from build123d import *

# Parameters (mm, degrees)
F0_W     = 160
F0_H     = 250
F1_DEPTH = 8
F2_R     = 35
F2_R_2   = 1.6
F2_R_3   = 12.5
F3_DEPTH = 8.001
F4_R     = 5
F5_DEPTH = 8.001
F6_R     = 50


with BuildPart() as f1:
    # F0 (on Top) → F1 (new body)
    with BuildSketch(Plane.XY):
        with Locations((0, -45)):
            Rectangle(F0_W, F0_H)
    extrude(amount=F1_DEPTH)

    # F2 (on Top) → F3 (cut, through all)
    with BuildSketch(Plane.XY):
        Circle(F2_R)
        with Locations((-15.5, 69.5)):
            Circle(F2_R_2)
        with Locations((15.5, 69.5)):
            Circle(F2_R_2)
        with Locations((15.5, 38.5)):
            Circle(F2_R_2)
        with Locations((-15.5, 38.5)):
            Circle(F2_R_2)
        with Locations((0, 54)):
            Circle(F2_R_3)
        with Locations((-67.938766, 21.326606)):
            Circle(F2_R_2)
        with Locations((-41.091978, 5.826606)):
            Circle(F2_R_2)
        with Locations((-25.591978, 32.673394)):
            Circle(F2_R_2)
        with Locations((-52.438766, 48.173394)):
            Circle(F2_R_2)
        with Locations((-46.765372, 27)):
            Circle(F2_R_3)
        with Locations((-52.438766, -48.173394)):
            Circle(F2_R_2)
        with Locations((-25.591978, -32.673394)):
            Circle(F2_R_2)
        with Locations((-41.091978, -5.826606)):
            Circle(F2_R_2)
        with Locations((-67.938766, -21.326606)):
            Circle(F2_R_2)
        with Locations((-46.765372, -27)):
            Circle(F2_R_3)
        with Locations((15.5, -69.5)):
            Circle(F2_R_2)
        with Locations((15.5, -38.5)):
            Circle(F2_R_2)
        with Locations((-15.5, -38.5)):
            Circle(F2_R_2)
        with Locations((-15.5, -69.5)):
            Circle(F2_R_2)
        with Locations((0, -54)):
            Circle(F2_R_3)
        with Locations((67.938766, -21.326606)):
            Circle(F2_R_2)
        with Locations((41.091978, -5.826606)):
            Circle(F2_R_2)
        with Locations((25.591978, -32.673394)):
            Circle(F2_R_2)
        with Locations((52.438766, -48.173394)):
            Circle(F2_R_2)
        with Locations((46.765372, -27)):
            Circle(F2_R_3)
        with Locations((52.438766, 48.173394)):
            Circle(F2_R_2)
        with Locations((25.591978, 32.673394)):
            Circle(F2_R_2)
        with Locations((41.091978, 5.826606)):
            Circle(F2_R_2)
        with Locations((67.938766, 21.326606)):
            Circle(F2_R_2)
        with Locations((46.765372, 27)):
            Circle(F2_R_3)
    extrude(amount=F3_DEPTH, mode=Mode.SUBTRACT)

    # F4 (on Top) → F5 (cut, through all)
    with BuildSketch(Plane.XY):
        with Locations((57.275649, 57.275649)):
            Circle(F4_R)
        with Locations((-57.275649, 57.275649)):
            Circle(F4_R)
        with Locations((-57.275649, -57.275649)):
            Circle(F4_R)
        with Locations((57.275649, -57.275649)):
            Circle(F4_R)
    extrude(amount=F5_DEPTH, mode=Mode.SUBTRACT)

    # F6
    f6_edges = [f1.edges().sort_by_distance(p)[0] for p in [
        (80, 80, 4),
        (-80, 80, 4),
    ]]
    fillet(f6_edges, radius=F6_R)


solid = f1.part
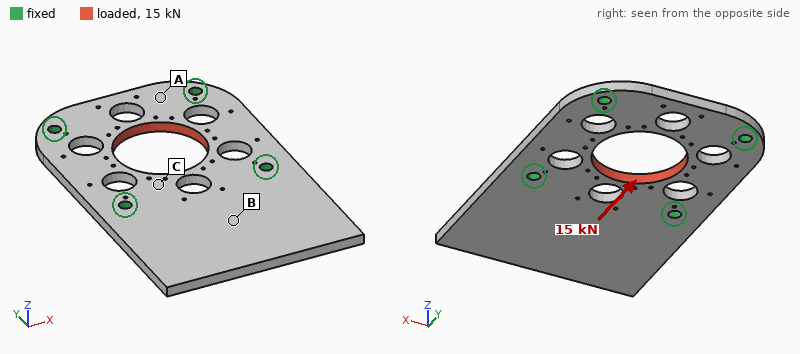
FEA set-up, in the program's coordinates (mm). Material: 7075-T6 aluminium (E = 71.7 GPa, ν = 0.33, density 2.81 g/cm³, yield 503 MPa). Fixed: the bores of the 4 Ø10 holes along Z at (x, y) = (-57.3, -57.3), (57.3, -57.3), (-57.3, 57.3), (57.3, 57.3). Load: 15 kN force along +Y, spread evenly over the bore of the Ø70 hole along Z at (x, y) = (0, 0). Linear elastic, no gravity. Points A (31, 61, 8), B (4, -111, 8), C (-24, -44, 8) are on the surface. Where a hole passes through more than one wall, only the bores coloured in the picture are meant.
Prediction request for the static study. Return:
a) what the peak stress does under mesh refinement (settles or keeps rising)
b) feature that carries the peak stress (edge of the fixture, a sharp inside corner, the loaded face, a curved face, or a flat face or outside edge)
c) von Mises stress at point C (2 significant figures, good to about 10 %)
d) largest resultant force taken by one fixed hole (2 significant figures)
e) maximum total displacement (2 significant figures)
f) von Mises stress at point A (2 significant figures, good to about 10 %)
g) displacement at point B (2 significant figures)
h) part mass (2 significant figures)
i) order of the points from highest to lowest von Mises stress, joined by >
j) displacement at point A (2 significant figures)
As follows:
keeps rising
edge of the fixture
8.3 MPa
4.0 kN
29 µm
12 MPa
5.8 µm
710 g
A > C > B
14 µm
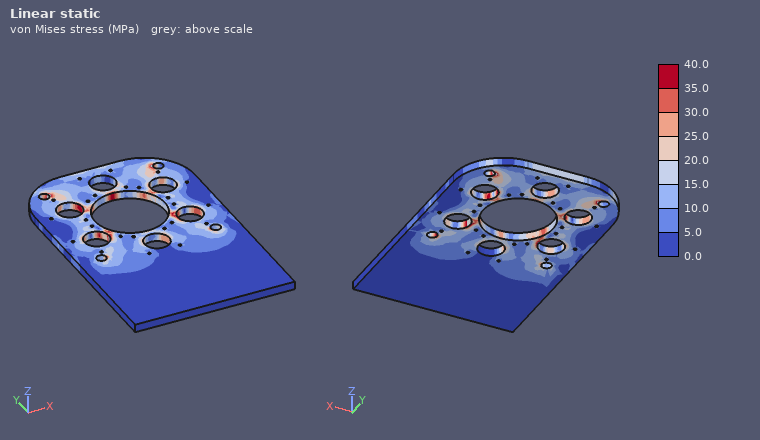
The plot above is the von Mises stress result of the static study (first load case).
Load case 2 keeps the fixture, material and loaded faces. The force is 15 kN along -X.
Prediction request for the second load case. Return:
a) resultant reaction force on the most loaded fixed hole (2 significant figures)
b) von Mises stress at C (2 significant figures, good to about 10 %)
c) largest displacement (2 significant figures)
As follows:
4.0 kN
17 MPa
30 µm
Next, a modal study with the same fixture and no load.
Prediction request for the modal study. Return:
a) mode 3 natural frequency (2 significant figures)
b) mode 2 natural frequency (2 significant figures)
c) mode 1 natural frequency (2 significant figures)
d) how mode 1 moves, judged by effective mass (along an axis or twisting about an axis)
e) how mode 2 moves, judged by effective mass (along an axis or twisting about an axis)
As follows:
2200 Hz
990 Hz
470 Hz
along Z
twisting about Y
